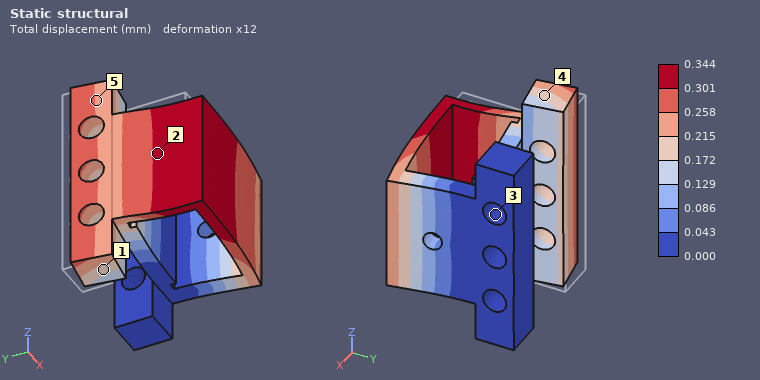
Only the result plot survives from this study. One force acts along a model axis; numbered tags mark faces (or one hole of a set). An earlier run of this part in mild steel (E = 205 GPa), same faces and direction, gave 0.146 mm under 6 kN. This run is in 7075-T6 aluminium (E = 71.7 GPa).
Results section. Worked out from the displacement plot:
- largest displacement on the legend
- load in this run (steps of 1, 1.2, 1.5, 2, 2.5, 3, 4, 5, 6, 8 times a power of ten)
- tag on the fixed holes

0.344 mm
5 kN
3
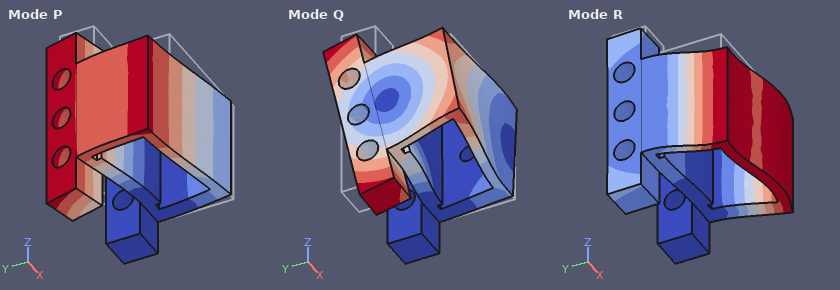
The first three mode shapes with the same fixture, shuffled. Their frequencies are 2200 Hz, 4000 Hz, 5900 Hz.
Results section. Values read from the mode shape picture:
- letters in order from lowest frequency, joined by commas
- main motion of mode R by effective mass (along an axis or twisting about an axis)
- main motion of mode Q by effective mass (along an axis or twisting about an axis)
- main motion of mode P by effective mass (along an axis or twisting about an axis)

P, Q, R
along X
twisting about X
along Y
